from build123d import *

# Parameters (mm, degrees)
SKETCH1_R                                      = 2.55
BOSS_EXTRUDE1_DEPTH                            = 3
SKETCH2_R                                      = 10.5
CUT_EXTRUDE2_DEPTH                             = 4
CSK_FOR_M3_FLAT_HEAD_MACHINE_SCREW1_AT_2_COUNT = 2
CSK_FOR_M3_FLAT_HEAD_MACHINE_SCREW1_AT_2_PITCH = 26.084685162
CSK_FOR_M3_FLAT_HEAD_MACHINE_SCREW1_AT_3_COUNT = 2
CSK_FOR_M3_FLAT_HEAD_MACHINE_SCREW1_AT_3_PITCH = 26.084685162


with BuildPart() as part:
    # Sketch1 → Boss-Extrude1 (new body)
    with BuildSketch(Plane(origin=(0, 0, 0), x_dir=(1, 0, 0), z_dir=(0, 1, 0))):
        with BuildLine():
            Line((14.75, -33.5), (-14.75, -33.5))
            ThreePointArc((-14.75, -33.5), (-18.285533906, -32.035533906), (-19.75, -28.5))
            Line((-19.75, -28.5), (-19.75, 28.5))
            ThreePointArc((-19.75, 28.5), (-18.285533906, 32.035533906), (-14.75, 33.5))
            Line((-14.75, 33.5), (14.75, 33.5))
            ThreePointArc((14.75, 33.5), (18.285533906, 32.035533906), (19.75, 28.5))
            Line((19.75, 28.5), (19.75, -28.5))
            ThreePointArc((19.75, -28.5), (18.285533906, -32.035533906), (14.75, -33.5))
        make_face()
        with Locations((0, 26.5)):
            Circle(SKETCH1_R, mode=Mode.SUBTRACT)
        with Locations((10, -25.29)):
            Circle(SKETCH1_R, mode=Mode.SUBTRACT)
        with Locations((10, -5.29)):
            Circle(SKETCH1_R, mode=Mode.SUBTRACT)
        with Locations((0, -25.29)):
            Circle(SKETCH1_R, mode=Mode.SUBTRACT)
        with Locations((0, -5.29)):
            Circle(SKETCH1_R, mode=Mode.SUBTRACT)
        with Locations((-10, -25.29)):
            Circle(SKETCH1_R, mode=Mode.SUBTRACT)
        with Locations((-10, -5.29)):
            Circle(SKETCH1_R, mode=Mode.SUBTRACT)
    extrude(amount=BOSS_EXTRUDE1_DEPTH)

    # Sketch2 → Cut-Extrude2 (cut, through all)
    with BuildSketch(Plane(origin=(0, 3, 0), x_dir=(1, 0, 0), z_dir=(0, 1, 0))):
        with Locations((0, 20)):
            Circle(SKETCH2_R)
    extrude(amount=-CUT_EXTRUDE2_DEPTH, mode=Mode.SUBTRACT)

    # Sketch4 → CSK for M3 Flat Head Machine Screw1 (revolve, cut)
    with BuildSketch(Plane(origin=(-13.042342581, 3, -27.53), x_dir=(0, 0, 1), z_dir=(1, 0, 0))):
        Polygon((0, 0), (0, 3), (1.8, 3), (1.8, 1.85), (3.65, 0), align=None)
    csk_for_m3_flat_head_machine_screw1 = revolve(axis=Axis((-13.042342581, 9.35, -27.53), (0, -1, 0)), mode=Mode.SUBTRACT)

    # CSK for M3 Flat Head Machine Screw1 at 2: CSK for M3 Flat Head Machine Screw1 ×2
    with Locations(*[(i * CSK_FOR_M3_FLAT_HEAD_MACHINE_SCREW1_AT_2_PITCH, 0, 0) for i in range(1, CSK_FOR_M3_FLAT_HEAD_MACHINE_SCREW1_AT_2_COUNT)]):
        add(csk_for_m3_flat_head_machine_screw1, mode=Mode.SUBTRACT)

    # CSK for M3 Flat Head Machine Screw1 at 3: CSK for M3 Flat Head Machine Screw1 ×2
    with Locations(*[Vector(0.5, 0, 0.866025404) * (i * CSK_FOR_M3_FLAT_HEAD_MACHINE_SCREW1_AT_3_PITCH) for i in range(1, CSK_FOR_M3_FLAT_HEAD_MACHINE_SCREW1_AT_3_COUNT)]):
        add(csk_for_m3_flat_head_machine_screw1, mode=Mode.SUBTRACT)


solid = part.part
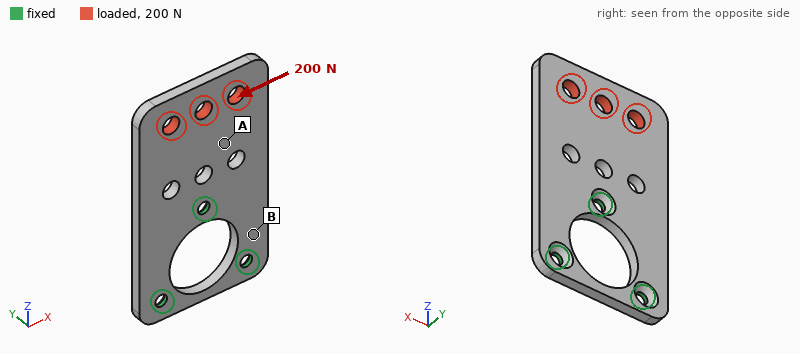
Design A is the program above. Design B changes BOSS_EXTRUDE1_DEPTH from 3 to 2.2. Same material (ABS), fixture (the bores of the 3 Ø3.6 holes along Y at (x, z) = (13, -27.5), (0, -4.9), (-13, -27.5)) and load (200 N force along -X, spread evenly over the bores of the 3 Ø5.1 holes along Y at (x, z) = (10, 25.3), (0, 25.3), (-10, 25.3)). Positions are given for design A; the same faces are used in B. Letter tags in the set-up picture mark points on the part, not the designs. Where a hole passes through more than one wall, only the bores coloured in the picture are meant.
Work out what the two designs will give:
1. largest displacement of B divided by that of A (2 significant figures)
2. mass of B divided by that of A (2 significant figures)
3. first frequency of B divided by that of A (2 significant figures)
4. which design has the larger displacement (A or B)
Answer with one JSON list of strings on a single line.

["1.3", "0.74", "0.79", "B"]
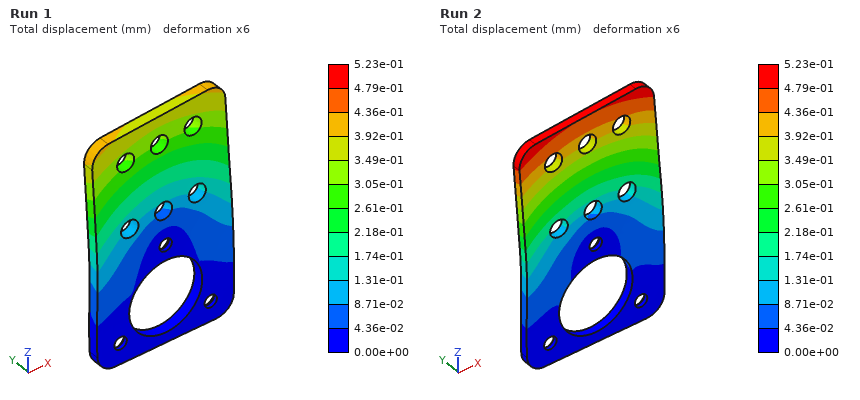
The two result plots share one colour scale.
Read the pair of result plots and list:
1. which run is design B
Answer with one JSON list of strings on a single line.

["Run 2"]
